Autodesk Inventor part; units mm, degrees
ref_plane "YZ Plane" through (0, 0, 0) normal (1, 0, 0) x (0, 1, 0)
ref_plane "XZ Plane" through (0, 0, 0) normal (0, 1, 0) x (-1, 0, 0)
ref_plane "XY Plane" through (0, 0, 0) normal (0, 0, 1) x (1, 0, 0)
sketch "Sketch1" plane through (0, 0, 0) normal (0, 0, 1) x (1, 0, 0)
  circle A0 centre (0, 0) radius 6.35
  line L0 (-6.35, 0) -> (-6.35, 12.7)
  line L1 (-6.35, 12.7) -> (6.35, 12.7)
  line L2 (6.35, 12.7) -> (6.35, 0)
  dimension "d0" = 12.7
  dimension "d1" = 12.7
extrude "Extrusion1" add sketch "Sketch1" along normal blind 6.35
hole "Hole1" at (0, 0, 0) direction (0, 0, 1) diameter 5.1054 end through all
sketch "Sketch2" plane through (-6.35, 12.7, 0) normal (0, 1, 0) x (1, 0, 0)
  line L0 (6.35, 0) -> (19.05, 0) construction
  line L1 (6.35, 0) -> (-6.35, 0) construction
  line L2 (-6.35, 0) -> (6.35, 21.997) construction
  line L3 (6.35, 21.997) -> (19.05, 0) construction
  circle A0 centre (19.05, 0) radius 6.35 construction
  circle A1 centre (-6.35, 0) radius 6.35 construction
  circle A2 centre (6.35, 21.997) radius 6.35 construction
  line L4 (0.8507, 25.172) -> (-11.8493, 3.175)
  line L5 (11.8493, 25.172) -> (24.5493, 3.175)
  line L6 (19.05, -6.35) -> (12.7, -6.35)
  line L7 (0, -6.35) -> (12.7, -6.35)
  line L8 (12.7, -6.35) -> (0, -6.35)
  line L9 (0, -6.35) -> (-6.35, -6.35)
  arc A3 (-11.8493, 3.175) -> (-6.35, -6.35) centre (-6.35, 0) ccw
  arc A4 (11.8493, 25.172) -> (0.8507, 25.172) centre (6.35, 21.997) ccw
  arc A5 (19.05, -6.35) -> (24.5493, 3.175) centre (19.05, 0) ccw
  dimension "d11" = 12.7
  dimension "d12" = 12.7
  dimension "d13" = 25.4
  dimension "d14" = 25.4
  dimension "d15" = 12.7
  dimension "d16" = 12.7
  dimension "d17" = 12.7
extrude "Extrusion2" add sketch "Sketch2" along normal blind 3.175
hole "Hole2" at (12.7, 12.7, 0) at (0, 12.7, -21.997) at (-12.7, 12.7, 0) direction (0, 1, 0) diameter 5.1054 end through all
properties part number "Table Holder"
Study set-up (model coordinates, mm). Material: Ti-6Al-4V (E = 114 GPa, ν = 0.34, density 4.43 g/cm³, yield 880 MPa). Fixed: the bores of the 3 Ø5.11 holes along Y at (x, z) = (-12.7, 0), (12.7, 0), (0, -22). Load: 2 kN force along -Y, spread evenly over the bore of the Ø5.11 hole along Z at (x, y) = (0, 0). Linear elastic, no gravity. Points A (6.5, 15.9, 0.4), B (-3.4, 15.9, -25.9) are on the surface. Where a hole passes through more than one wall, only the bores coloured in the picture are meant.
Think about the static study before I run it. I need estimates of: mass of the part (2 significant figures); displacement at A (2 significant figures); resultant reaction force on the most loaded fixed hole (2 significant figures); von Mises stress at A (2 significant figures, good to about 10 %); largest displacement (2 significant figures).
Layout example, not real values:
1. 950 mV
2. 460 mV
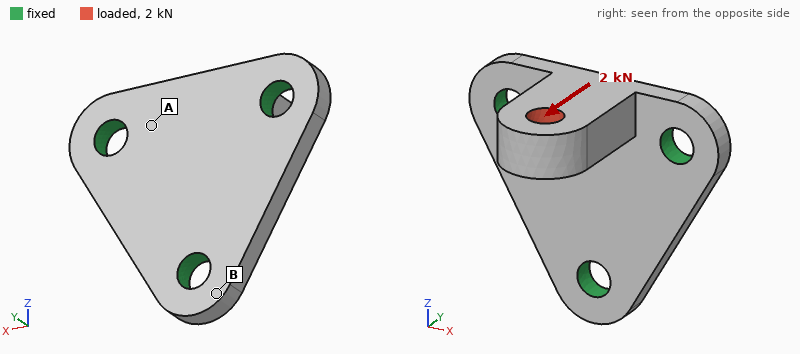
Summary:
1. 17 g
2. 9.2 µm
3. 1.1 kN
4. 62 MPa
5. 56 µm
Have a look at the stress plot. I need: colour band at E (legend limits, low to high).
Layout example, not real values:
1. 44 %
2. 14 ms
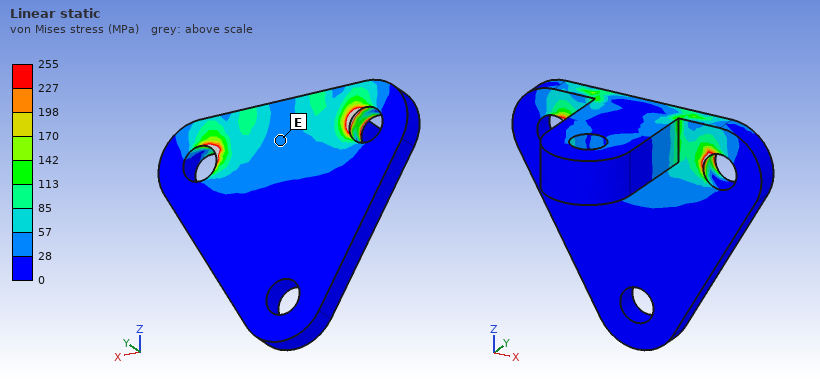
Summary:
1. 28 to 57 MPa
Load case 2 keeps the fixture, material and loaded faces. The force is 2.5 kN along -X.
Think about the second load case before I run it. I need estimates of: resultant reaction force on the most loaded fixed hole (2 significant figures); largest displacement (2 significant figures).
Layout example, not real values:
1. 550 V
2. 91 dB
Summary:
1. 2.4 kN
2. 0.11 mm
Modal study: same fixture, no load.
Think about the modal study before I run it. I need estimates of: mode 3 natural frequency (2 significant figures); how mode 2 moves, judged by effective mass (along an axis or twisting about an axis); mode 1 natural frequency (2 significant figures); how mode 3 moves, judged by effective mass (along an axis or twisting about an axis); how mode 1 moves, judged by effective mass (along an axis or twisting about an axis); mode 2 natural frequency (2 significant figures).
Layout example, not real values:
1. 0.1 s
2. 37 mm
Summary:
1. 21 kHz
2. along X
3. 7200 Hz
4. along Y
5. along Z
6. 15 kHz
